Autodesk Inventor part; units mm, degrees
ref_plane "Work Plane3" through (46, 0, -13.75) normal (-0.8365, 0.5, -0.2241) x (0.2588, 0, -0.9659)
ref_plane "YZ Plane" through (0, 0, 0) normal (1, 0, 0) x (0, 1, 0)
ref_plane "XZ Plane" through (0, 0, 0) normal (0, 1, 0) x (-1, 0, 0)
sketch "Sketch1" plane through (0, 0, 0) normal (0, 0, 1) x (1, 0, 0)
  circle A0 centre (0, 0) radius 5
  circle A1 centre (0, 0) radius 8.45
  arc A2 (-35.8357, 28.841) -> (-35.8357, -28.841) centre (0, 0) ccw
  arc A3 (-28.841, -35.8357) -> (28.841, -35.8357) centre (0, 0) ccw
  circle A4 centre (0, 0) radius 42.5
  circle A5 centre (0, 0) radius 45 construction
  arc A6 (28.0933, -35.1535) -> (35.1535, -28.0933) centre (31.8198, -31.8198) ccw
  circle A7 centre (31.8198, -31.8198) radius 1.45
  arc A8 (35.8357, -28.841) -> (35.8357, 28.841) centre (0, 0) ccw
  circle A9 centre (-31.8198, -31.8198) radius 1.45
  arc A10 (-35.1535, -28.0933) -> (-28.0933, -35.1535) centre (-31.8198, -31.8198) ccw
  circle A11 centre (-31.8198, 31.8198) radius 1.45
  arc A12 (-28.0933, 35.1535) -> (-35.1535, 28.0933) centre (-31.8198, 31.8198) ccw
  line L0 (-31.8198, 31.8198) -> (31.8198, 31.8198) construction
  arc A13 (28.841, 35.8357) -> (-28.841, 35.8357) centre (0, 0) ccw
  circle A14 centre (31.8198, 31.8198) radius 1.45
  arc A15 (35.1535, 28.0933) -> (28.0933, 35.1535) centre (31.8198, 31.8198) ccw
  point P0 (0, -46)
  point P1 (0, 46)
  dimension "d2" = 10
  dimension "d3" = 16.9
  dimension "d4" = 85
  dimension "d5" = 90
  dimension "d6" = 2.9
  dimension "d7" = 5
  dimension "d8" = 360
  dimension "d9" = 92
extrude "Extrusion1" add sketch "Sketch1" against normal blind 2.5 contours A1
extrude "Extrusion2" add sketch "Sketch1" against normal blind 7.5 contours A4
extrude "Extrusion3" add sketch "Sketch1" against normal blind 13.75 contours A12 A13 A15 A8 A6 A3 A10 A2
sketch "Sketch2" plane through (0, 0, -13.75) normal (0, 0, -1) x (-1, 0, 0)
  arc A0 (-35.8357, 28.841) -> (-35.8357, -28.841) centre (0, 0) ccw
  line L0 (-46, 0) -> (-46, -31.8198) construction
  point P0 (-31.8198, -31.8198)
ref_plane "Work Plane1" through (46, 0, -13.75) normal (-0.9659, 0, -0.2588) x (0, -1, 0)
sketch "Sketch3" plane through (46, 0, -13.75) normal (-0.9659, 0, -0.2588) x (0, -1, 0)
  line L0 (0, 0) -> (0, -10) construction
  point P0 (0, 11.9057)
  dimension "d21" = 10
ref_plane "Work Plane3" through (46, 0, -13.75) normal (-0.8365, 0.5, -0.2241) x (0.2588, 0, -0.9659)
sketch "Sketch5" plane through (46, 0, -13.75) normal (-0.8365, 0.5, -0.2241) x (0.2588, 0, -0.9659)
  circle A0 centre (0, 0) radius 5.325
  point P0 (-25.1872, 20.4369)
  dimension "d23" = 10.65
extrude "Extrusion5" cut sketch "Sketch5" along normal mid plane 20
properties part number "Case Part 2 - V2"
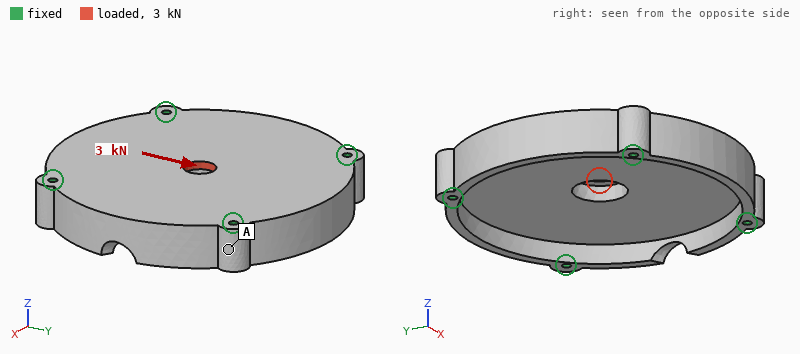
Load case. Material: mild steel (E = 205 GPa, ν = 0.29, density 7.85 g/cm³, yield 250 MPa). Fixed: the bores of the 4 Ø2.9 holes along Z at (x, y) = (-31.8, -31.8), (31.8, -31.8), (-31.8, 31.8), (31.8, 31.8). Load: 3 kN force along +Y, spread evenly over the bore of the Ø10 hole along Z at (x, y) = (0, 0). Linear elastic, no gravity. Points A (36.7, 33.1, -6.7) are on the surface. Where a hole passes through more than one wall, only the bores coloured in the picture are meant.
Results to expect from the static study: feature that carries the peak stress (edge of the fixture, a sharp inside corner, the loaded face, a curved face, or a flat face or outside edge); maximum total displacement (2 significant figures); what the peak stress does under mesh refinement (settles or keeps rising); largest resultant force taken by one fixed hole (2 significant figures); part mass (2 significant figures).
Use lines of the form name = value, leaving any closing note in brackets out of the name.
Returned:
feature that carries the peak stress = a sharp inside corner
maximum total displacement = 2.9 µm
what the peak stress does under mesh refinement = keeps rising
largest resultant force taken by one fixed hole = 790 N
part mass = 440 g
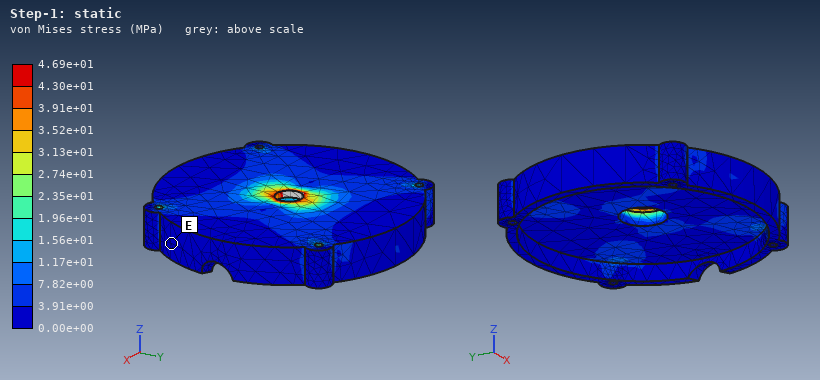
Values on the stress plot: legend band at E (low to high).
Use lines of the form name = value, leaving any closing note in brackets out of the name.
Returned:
legend band at E = 0.00e+00 to 3.91e+00 MPa
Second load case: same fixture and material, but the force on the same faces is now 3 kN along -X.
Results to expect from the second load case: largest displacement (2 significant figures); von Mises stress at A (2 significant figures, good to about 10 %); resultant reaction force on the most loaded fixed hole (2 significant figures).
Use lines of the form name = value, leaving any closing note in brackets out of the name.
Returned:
largest displacement = 2.9 µm
von Mises stress at A = 3.5 MPa
resultant reaction force on the most loaded fixed hole = 790 N
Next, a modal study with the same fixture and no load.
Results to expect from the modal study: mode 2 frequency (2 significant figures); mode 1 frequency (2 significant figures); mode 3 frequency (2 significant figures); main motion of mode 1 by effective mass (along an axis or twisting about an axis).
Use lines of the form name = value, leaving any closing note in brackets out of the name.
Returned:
mode 2 frequency = 9800 Hz
mode 1 frequency = 6200 Hz
mode 3 frequency = 9900 Hz
main motion of mode 1 by effective mass = along Z
